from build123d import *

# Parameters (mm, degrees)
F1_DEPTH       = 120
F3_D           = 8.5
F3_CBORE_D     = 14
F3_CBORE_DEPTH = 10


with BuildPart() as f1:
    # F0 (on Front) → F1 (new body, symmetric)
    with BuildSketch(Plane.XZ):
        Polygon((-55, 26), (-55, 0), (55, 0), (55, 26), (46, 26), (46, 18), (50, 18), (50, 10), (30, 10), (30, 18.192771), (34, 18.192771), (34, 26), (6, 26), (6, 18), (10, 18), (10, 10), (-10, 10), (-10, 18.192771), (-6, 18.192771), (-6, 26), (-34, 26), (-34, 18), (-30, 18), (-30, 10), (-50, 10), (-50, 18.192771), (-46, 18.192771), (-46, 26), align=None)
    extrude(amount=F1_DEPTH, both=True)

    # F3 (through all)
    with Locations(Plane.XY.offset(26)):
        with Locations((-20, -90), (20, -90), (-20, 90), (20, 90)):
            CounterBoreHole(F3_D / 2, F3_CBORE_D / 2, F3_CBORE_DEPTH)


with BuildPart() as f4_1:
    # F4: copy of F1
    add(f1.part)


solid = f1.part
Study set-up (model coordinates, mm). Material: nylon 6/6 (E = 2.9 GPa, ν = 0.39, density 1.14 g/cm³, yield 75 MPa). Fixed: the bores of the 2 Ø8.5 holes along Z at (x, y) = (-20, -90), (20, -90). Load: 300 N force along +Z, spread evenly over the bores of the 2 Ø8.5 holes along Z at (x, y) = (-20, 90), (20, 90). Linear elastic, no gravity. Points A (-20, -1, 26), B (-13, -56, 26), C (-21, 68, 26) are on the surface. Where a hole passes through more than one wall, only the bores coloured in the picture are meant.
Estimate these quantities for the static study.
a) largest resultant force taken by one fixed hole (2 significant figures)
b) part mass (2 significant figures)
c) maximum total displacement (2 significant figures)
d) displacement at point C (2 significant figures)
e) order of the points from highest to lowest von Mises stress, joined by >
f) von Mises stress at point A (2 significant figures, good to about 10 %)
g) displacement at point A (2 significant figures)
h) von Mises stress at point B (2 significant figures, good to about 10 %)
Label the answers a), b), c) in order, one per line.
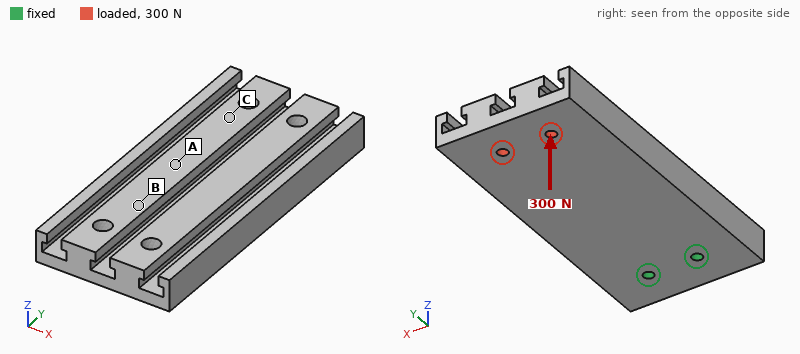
a) 240 N
b) 560 g
c) 3.1 mm
d) 2.1 mm
e) B > A > C
f) 3.1 MPa
g) 0.97 mm
h) 5.1 MPa
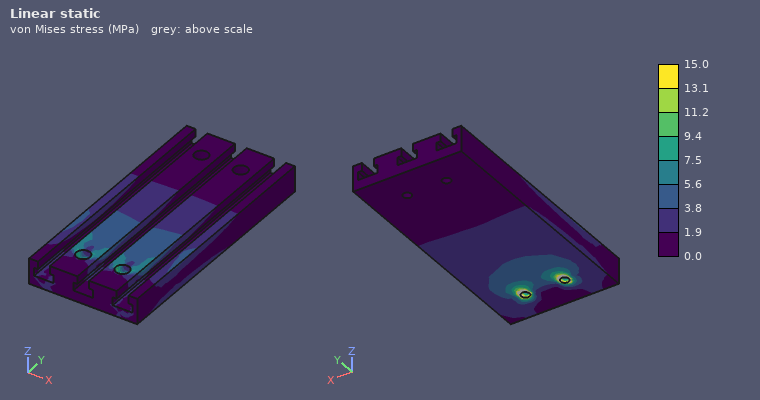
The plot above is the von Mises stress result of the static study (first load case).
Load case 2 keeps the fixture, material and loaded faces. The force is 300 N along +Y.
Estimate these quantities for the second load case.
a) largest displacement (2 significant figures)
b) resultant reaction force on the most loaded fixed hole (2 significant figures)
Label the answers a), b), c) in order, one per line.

a) 62 µm
b) 150 N
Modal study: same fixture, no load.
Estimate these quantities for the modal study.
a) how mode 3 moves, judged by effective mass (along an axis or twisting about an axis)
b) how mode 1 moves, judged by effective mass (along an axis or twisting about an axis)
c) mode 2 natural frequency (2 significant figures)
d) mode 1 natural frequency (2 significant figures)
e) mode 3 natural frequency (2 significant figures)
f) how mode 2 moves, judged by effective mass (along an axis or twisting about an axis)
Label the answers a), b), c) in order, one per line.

a) along X
b) along Z
c) 290 Hz
d) 120 Hz
e) 360 Hz
f) along X
